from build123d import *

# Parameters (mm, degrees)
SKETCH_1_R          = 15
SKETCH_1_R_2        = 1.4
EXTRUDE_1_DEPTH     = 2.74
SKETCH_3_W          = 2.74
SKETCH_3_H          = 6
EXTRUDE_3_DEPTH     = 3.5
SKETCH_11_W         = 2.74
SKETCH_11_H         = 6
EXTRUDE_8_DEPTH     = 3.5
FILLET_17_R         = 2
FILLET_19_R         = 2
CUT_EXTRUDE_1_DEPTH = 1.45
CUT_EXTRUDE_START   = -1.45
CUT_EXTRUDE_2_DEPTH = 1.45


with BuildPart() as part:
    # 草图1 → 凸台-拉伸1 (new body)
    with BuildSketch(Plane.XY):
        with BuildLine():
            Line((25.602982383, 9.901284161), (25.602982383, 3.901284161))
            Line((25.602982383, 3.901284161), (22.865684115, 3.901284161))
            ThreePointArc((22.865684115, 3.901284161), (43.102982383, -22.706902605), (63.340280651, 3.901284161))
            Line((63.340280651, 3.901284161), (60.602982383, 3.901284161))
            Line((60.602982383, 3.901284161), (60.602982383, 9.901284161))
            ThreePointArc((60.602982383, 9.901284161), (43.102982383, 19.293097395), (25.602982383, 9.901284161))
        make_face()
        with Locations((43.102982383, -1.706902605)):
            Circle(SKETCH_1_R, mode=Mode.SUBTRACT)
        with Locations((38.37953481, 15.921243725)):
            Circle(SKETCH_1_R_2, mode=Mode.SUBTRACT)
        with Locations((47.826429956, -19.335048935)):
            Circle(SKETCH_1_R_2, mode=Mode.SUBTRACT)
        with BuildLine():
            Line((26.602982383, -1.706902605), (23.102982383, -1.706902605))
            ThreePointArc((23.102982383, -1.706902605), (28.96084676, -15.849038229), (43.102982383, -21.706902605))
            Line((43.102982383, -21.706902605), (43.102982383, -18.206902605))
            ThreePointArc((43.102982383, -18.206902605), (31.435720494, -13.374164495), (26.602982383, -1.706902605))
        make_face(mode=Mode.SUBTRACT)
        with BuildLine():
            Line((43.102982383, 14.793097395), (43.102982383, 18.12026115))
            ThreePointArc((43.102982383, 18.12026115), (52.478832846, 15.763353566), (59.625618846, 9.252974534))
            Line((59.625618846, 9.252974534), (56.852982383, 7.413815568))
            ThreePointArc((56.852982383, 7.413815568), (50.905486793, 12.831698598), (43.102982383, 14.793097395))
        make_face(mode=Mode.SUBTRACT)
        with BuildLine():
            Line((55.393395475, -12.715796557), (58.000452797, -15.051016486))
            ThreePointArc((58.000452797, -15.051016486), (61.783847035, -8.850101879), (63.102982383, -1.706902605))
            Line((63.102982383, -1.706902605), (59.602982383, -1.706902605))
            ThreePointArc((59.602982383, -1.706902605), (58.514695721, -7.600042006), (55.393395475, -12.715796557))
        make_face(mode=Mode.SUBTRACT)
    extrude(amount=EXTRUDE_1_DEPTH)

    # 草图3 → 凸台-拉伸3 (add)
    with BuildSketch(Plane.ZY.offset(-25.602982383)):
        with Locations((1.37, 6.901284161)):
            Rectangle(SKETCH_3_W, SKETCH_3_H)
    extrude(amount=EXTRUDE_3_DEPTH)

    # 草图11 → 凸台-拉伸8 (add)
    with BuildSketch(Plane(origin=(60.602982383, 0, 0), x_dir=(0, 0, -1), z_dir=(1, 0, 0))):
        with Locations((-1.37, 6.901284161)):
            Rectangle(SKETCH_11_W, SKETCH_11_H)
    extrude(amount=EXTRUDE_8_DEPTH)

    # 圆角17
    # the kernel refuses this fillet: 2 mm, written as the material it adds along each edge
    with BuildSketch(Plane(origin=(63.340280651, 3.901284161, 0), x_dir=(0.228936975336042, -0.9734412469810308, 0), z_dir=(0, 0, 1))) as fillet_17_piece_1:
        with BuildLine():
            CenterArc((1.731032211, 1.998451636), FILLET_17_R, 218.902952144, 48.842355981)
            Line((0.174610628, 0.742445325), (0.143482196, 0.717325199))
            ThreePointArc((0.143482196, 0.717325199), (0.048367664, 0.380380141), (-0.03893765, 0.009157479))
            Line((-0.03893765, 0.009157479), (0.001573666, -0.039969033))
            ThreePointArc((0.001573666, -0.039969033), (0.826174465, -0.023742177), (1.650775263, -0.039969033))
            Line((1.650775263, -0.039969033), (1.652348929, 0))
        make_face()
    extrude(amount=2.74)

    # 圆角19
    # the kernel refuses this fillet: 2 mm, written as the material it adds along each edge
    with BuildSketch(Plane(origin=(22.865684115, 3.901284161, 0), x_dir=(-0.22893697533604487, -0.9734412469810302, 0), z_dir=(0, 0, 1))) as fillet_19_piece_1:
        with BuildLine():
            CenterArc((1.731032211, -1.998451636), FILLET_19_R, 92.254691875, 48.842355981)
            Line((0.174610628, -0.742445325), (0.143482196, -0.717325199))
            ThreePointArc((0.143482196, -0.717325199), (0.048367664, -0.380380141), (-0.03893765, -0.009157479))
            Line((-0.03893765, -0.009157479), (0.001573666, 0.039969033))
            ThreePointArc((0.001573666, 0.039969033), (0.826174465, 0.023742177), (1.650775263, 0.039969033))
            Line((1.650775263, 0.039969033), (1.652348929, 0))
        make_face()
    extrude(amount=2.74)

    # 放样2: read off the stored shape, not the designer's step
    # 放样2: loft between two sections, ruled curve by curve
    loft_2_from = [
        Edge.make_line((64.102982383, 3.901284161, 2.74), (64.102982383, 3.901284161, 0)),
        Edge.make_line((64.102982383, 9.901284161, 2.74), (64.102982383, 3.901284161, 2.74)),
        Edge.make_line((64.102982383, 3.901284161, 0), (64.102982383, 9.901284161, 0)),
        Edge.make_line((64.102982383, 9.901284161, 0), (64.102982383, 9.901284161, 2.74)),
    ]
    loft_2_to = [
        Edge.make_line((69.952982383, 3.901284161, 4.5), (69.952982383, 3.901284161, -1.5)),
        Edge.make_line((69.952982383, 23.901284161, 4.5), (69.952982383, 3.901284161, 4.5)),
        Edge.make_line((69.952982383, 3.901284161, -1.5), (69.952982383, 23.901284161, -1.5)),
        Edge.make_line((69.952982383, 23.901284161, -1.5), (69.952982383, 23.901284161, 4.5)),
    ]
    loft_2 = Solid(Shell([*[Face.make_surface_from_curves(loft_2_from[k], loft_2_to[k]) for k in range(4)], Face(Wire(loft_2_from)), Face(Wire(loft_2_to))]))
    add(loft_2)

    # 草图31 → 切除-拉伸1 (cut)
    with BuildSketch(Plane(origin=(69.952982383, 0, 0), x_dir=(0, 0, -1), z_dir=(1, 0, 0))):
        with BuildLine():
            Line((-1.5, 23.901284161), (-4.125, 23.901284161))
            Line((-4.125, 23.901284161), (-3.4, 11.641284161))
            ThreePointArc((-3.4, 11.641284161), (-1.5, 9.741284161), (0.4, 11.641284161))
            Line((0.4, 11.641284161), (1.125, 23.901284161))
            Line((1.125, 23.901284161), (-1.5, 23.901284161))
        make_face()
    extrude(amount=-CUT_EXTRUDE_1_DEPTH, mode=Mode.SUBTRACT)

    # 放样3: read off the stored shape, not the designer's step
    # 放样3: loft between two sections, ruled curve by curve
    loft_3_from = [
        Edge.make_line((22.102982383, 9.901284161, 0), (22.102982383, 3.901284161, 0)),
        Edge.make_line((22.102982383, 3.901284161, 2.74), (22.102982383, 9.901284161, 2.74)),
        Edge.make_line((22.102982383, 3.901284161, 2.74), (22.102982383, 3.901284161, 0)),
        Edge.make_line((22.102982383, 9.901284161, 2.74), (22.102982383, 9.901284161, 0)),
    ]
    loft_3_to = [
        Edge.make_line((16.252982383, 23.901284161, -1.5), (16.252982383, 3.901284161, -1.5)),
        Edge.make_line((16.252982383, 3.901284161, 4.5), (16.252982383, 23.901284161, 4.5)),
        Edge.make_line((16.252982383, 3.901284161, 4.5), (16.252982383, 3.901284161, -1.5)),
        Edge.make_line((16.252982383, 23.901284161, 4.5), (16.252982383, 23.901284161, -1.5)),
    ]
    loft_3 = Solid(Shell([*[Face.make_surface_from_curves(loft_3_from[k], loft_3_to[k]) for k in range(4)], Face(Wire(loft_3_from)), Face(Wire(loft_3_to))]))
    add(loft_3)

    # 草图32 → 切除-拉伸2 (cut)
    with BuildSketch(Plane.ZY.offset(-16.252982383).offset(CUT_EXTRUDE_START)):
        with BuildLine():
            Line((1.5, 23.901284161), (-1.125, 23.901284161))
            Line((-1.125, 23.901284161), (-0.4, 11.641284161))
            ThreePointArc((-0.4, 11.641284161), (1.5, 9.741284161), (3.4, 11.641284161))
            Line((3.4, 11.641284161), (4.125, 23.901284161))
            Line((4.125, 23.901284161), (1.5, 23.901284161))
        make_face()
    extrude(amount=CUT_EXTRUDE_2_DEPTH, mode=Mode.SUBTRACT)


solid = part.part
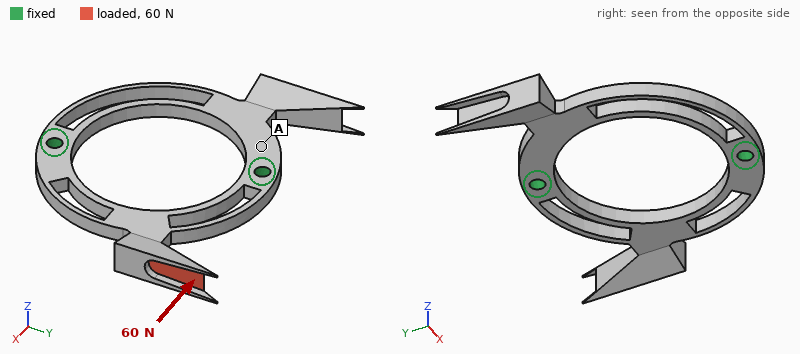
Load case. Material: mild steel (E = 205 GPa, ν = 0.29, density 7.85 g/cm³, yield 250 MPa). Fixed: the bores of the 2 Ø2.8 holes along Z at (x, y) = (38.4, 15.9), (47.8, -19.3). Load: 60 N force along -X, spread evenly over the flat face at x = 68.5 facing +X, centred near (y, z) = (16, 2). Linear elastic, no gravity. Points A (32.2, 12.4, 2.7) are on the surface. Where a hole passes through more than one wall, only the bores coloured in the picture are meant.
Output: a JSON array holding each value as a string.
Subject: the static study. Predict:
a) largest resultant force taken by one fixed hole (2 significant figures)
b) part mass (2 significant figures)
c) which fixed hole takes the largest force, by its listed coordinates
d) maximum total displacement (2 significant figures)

["68 N", "15 g", "(38.4, 15.9)", "36 µm"]
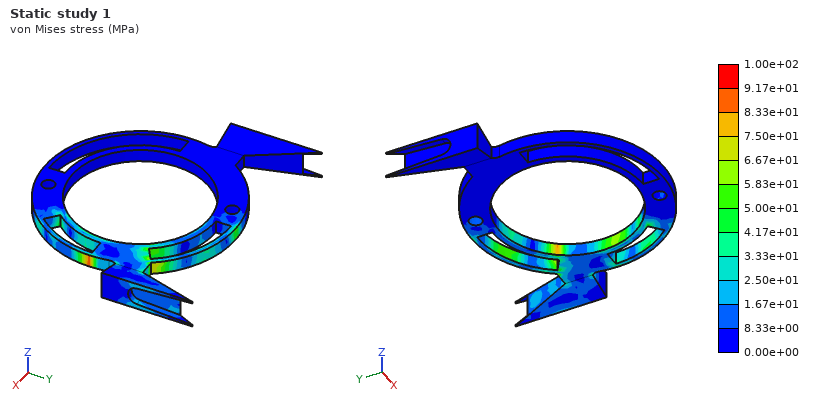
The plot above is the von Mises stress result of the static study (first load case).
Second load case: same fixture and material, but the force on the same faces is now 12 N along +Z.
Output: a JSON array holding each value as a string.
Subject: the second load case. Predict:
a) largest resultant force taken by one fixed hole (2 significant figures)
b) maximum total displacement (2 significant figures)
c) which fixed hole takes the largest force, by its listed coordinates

["9.5 N", "89 µm", "(38.4, 15.9)"]
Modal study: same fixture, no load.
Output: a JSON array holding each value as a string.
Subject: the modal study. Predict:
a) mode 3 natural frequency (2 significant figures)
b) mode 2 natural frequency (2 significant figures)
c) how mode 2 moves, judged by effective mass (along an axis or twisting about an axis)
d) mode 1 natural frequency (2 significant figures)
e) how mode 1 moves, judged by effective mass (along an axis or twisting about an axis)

["5700 Hz", "2600 Hz", "along Z", "1500 Hz", "along Z"]
